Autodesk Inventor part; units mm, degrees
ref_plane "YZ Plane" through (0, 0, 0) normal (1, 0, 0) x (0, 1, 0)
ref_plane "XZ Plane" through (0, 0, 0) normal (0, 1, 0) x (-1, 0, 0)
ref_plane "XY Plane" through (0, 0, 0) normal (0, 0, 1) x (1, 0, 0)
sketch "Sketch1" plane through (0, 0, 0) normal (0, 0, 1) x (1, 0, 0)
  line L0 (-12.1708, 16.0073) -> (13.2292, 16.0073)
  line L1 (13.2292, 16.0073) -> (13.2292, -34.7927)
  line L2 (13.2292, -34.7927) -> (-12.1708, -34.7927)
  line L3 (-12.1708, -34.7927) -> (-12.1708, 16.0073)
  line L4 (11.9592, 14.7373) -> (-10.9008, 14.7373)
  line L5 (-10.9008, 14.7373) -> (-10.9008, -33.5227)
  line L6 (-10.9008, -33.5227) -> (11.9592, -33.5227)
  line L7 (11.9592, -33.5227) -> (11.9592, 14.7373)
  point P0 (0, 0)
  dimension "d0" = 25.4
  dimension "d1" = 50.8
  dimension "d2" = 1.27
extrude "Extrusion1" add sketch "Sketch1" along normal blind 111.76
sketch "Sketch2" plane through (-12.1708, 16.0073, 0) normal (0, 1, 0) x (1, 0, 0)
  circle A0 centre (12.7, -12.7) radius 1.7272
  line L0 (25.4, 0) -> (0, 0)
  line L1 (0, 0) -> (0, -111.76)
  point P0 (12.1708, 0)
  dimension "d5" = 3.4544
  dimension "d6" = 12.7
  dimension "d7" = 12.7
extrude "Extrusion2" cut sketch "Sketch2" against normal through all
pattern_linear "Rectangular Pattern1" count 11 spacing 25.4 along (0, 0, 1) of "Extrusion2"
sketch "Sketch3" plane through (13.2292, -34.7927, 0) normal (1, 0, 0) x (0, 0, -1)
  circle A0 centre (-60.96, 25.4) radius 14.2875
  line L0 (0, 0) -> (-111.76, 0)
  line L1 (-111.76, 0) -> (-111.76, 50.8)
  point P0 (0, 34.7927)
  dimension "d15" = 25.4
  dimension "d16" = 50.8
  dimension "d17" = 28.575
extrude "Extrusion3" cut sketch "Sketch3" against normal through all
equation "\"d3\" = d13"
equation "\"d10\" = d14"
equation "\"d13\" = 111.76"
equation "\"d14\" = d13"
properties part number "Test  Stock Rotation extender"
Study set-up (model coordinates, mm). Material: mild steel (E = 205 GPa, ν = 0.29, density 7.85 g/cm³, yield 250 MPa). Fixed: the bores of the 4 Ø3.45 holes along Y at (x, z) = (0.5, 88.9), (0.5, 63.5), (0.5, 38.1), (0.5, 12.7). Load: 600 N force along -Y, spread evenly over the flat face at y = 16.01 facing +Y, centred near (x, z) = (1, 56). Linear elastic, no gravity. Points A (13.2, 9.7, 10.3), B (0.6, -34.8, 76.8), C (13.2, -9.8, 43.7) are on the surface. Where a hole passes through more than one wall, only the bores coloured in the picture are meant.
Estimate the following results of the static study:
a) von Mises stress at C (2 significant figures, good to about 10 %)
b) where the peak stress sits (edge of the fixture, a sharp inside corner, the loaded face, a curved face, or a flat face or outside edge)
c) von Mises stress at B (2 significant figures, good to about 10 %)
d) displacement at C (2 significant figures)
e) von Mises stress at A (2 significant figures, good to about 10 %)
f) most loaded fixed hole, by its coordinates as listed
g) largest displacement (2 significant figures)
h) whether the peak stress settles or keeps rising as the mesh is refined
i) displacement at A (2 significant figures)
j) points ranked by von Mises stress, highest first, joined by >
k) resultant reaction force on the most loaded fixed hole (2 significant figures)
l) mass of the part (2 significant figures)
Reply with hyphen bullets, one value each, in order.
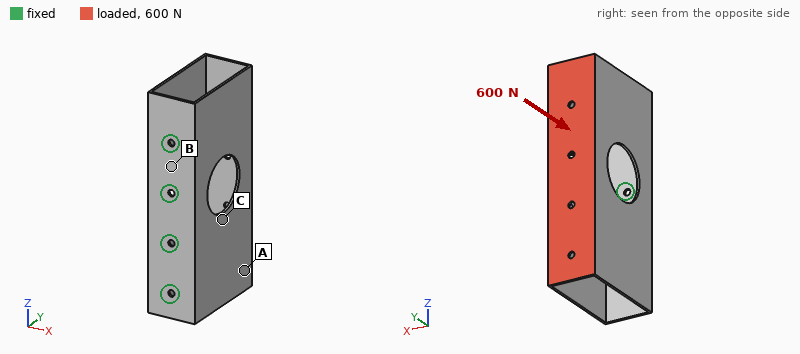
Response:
- 17 MPa
- edge of the fixture
- 67 MPa
- 53 µm
- 8.9 MPa
- (0.5, 88.9)
- 63 µm
- keeps rising
- 29 µm
- B > C > A
- 200 N
- 150 g
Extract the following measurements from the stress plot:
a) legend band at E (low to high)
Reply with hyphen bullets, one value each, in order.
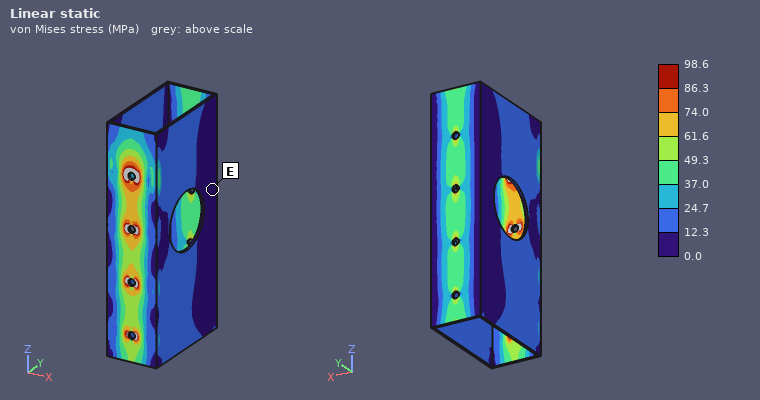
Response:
- 0.0 to 12.3 MPa
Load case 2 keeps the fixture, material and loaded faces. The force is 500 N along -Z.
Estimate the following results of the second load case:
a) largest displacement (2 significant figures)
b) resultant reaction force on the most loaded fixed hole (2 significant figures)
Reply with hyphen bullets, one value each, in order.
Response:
- 0.11 mm
- 310 N
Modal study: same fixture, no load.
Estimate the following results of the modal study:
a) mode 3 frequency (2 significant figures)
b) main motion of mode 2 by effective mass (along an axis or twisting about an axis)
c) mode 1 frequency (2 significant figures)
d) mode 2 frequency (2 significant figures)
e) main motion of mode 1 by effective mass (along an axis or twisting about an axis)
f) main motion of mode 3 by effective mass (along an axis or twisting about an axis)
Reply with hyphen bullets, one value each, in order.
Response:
- 1200 Hz
- twisting about Y
- 310 Hz
- 1000 Hz
- along X
- along Z
